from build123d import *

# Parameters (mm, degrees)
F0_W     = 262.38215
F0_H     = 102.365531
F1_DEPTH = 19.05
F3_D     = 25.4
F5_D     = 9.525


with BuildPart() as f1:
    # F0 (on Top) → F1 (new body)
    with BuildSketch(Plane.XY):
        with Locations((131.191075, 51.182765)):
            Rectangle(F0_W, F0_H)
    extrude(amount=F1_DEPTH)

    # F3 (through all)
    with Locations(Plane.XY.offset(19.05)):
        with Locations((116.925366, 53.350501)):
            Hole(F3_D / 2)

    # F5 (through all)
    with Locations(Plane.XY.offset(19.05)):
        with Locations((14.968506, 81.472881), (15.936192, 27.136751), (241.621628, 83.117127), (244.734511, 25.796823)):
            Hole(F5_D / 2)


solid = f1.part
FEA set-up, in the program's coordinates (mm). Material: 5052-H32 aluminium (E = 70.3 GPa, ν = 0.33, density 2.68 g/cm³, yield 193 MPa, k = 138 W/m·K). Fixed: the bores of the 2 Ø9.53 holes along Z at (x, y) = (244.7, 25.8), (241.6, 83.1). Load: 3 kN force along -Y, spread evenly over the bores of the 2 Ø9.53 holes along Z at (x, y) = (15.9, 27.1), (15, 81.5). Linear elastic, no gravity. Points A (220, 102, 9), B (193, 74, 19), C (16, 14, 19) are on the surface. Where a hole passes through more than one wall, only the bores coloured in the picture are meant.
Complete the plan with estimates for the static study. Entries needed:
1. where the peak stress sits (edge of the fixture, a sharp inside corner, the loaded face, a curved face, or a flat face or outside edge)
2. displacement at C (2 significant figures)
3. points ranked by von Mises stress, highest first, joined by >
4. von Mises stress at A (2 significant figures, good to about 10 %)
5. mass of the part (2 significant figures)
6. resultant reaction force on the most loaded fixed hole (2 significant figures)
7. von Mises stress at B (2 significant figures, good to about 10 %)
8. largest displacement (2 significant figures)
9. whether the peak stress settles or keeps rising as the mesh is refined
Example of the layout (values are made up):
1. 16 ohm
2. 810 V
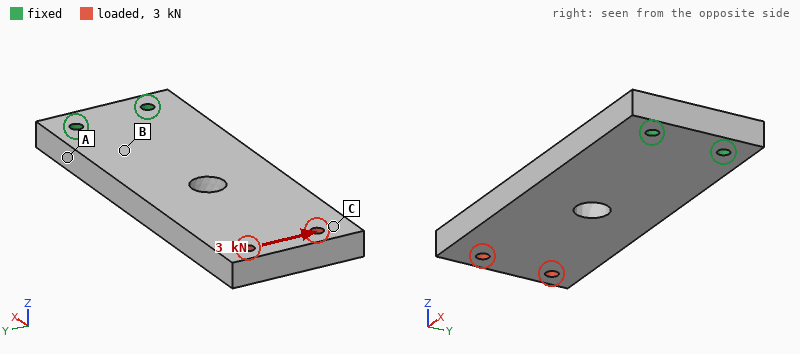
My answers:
1. edge of the fixture
2. 0.14 mm
3. A > B > C
4. 16 MPa
5. 1.3 kg
6. 11 kN
7. 8.4 MPa
8. 0.15 mm
9. keeps rising
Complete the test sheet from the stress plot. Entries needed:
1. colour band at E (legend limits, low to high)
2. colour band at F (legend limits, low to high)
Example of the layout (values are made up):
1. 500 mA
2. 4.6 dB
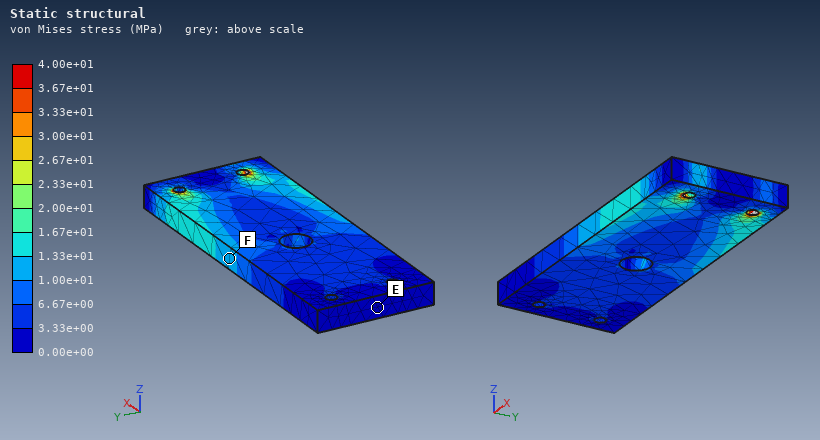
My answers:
1. 0.00e+00 to 3.33e+00 MPa
2. 1.00e+01 to 1.33e+01 MPa
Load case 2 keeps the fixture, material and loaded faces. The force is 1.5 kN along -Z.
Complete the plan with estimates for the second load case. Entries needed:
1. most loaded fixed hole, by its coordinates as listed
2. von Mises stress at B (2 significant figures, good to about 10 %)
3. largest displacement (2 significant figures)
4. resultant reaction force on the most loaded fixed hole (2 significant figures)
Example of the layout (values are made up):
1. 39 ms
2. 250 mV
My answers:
1. (241.6, 83.1)
2. 42 MPa
3. 1.7 mm
4. 940 N
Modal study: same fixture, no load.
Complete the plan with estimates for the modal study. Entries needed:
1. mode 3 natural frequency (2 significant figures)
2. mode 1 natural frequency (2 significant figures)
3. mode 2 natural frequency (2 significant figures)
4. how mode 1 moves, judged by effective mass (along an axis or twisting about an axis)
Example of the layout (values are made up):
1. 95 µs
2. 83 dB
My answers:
1. 1200 Hz
2. 260 Hz
3. 1200 Hz
4. along Z
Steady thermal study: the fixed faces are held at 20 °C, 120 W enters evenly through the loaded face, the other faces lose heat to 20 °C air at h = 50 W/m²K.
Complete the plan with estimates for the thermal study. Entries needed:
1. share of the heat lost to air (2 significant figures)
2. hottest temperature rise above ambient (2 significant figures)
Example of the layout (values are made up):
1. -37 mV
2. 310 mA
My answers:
1. 66 %
2. 60 K
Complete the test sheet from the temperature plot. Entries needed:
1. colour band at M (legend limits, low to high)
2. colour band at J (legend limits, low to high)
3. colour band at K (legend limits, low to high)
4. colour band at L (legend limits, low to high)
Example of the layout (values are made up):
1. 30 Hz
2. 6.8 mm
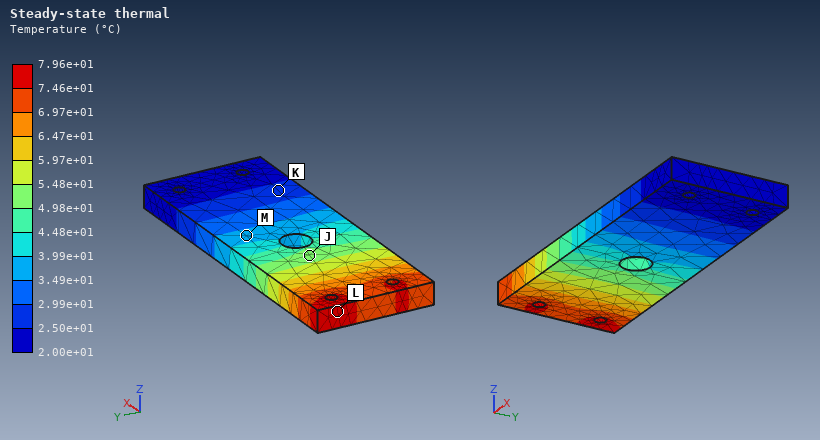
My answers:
1. 3.49e+01 to 3.99e+01 °C
2. 4.98e+01 to 5.48e+01 °C
3. 2.50e+01 to 2.99e+01 °C
4. 7.46e+01 to 7.96e+01 °C
